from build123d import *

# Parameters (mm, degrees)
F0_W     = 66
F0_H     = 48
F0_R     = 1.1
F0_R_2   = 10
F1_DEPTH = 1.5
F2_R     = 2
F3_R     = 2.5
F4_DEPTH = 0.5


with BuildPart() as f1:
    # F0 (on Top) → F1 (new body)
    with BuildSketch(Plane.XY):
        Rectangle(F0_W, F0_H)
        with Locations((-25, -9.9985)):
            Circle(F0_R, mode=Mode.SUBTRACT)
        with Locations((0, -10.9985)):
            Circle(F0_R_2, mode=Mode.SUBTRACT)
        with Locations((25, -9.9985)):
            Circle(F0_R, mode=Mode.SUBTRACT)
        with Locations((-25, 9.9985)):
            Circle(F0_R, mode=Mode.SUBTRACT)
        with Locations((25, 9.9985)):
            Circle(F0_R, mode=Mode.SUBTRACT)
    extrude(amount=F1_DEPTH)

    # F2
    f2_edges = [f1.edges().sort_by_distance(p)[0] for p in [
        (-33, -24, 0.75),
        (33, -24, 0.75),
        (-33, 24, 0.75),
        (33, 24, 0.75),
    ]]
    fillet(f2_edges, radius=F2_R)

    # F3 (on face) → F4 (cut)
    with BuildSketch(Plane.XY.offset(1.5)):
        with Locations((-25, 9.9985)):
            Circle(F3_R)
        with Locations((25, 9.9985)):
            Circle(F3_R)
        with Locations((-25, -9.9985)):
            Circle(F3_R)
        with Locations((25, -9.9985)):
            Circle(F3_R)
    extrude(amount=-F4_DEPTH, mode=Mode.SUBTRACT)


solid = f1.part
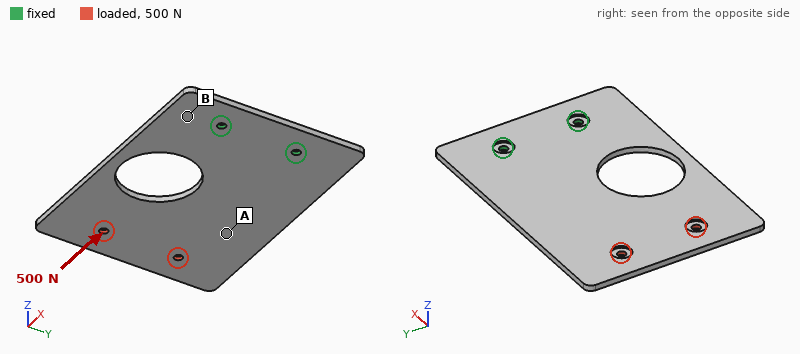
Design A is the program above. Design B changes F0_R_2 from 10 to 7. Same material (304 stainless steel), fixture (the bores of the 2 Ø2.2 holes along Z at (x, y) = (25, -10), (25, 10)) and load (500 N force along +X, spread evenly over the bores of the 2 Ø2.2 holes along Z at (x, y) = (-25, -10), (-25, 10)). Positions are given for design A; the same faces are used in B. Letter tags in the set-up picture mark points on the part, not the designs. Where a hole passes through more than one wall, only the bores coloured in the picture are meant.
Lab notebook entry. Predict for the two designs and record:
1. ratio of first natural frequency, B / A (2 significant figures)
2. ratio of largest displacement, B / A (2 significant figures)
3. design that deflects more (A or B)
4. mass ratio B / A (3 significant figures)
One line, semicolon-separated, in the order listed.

1.0; 0.85; A; 1.06
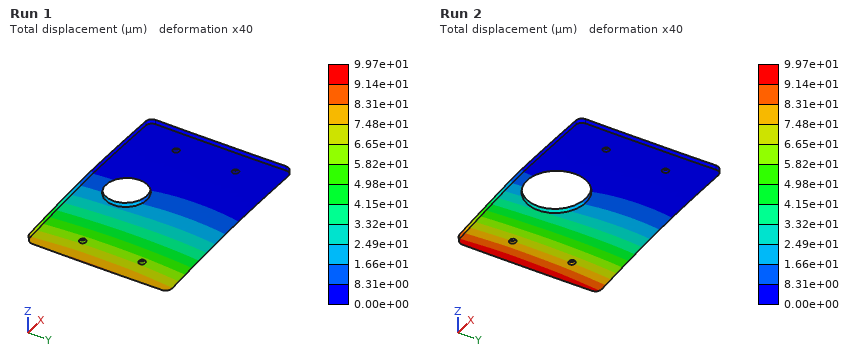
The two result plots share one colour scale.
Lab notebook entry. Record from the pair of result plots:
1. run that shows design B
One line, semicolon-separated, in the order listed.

Run 1
